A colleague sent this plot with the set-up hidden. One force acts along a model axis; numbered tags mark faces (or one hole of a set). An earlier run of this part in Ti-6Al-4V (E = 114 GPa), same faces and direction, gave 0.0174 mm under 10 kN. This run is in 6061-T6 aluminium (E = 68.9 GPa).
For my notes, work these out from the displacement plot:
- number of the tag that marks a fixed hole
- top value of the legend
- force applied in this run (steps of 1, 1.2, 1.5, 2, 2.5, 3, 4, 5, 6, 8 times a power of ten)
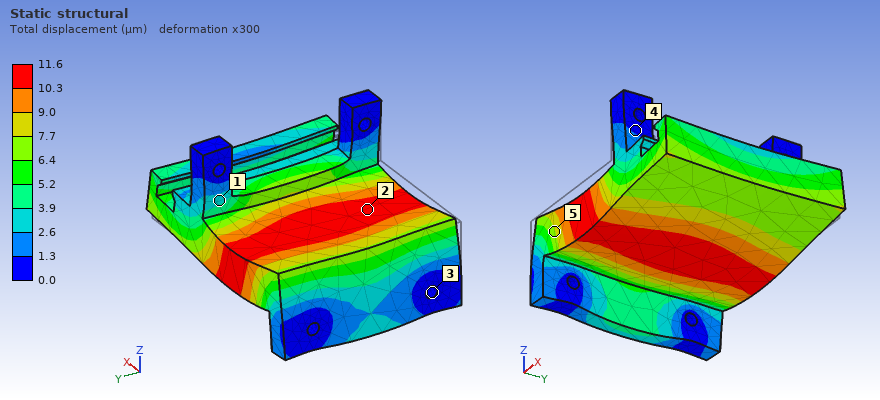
3
11.6 µm
4 kN
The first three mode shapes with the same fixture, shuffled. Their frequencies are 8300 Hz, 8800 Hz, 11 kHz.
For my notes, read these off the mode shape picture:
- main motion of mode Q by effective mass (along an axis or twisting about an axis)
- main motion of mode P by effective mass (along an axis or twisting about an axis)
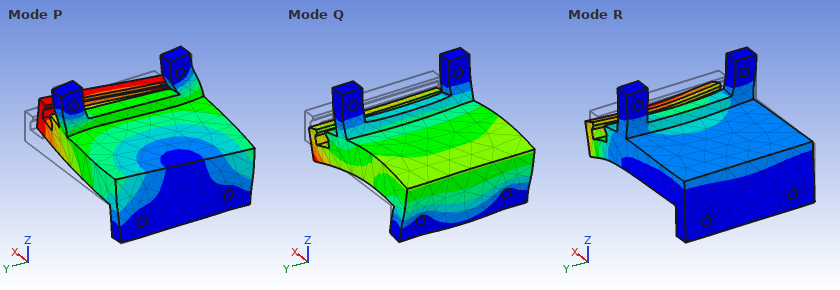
along X
along Y
